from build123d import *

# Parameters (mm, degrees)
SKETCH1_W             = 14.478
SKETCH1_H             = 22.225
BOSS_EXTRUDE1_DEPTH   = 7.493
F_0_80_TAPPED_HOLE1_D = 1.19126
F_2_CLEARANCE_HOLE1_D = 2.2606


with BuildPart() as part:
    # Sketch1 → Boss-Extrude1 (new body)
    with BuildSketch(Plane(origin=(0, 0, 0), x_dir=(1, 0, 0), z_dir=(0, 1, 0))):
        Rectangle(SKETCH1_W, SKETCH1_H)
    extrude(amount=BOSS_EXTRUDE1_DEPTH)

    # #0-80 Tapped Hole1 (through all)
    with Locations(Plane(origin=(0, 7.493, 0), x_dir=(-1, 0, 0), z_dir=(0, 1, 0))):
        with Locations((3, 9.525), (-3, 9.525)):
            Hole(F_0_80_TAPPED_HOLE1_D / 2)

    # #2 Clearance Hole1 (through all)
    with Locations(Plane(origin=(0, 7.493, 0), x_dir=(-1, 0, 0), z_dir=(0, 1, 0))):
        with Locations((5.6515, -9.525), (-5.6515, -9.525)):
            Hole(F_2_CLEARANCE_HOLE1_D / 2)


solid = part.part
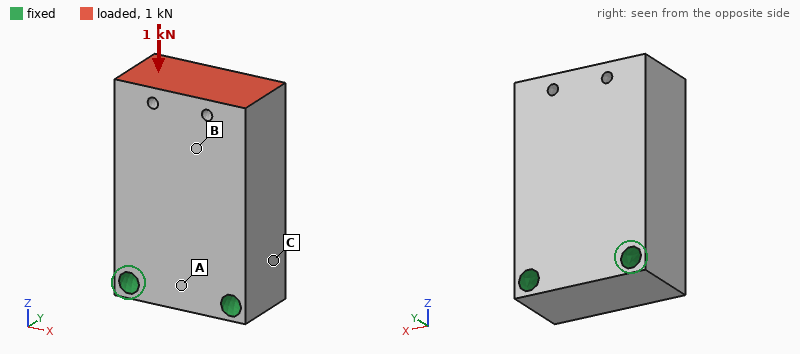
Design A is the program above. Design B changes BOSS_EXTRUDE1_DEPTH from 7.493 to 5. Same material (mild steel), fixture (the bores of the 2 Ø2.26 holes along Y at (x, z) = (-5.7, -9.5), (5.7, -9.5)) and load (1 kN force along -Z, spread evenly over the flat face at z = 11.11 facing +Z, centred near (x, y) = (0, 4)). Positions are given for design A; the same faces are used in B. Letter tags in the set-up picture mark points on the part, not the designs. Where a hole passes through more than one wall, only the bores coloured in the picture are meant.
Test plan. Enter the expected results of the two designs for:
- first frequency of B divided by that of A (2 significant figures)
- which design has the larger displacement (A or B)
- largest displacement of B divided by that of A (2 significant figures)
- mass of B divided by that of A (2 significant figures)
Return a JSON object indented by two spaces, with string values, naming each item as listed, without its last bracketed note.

{
  "first frequency of B divided by that of A": "0.71",
  "which design has the larger displacement": "B",
  "largest displacement of B divided by that of A": "1.5",
  "mass of B divided by that of A": "0.67"
}
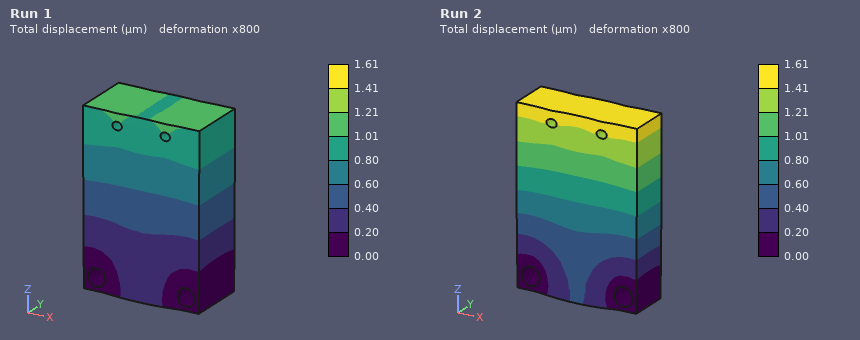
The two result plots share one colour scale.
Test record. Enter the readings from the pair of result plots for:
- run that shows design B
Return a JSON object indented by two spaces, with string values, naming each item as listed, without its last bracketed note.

{
  "run that shows design B": "Run 2"
}
